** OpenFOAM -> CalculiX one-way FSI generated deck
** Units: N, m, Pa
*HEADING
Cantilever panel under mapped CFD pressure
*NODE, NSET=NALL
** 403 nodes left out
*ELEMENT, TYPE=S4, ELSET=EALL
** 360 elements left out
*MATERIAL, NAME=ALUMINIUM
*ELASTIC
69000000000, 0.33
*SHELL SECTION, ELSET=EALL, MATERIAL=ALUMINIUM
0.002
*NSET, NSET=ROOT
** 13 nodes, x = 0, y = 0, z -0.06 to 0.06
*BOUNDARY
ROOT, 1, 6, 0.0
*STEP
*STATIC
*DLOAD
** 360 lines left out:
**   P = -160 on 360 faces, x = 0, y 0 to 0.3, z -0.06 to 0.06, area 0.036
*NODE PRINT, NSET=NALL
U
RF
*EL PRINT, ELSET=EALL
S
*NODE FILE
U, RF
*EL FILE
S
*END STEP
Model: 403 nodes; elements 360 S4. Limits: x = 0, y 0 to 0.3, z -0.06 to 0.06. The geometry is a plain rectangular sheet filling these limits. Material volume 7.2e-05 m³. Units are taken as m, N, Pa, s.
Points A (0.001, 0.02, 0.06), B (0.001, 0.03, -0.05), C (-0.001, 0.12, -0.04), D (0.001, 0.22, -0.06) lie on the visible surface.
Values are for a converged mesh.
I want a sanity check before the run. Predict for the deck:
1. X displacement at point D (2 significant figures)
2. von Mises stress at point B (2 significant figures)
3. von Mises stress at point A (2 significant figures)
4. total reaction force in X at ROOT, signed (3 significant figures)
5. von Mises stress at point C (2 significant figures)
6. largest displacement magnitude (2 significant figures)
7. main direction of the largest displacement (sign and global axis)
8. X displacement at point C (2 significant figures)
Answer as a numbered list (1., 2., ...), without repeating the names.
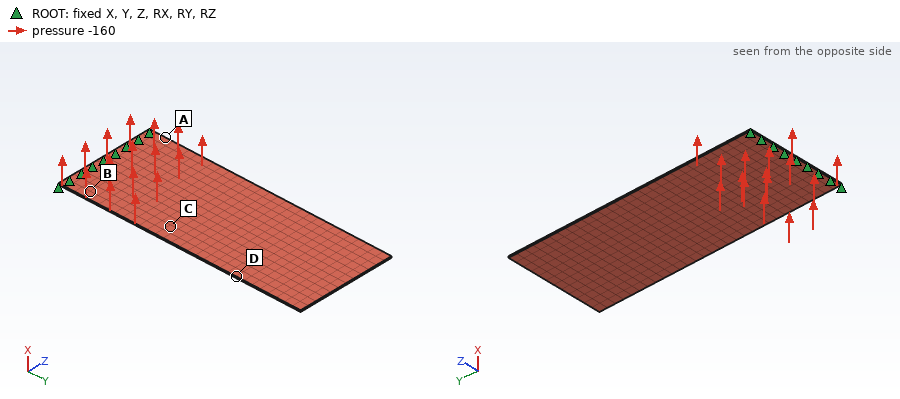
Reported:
1. 0.0021 m
2. 8.5e+06 Pa
3. 9.2e+06 Pa
4. -5.76 N
5. 3.9e+06 Pa
6. 0.0033 m
7. +X
8. 7.8e-04 m
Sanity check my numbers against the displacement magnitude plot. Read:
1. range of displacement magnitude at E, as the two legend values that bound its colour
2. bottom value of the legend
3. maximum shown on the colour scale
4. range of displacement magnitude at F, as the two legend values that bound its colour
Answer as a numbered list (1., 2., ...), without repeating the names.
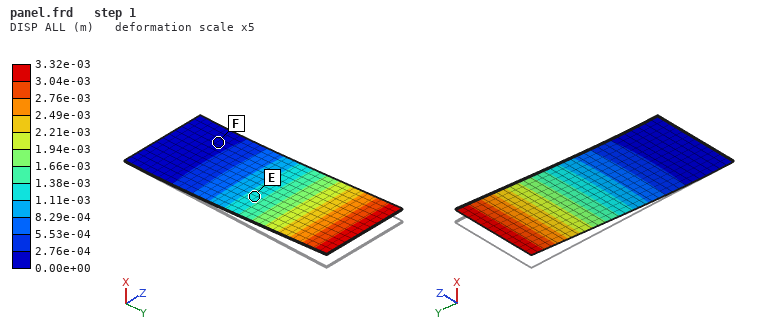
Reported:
1. 1.11e-03 to 1.38e-03 m
2. 0.00e+00 m
3. 3.32e-03 m
4. 0.00e+00 to 2.76e-04 m
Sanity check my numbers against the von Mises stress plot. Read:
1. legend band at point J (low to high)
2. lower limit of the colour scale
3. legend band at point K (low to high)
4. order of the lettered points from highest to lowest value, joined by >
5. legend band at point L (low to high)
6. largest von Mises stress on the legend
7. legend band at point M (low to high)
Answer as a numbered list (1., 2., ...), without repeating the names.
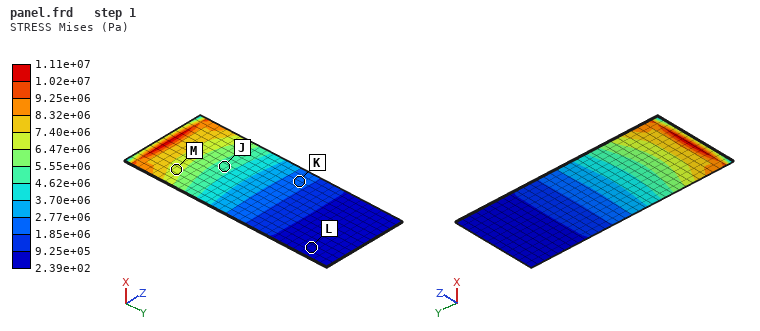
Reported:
1. 4.62e+06 to 5.55e+06 Pa
2. 2.39e+02 Pa
3. 1.85e+06 to 2.77e+06 Pa
4. M > J > K > L
5. 2.39e+02 to 9.25e+05 Pa
6. 1.11e+07 Pa
7. 6.47e+06 to 7.40e+06 Pa
